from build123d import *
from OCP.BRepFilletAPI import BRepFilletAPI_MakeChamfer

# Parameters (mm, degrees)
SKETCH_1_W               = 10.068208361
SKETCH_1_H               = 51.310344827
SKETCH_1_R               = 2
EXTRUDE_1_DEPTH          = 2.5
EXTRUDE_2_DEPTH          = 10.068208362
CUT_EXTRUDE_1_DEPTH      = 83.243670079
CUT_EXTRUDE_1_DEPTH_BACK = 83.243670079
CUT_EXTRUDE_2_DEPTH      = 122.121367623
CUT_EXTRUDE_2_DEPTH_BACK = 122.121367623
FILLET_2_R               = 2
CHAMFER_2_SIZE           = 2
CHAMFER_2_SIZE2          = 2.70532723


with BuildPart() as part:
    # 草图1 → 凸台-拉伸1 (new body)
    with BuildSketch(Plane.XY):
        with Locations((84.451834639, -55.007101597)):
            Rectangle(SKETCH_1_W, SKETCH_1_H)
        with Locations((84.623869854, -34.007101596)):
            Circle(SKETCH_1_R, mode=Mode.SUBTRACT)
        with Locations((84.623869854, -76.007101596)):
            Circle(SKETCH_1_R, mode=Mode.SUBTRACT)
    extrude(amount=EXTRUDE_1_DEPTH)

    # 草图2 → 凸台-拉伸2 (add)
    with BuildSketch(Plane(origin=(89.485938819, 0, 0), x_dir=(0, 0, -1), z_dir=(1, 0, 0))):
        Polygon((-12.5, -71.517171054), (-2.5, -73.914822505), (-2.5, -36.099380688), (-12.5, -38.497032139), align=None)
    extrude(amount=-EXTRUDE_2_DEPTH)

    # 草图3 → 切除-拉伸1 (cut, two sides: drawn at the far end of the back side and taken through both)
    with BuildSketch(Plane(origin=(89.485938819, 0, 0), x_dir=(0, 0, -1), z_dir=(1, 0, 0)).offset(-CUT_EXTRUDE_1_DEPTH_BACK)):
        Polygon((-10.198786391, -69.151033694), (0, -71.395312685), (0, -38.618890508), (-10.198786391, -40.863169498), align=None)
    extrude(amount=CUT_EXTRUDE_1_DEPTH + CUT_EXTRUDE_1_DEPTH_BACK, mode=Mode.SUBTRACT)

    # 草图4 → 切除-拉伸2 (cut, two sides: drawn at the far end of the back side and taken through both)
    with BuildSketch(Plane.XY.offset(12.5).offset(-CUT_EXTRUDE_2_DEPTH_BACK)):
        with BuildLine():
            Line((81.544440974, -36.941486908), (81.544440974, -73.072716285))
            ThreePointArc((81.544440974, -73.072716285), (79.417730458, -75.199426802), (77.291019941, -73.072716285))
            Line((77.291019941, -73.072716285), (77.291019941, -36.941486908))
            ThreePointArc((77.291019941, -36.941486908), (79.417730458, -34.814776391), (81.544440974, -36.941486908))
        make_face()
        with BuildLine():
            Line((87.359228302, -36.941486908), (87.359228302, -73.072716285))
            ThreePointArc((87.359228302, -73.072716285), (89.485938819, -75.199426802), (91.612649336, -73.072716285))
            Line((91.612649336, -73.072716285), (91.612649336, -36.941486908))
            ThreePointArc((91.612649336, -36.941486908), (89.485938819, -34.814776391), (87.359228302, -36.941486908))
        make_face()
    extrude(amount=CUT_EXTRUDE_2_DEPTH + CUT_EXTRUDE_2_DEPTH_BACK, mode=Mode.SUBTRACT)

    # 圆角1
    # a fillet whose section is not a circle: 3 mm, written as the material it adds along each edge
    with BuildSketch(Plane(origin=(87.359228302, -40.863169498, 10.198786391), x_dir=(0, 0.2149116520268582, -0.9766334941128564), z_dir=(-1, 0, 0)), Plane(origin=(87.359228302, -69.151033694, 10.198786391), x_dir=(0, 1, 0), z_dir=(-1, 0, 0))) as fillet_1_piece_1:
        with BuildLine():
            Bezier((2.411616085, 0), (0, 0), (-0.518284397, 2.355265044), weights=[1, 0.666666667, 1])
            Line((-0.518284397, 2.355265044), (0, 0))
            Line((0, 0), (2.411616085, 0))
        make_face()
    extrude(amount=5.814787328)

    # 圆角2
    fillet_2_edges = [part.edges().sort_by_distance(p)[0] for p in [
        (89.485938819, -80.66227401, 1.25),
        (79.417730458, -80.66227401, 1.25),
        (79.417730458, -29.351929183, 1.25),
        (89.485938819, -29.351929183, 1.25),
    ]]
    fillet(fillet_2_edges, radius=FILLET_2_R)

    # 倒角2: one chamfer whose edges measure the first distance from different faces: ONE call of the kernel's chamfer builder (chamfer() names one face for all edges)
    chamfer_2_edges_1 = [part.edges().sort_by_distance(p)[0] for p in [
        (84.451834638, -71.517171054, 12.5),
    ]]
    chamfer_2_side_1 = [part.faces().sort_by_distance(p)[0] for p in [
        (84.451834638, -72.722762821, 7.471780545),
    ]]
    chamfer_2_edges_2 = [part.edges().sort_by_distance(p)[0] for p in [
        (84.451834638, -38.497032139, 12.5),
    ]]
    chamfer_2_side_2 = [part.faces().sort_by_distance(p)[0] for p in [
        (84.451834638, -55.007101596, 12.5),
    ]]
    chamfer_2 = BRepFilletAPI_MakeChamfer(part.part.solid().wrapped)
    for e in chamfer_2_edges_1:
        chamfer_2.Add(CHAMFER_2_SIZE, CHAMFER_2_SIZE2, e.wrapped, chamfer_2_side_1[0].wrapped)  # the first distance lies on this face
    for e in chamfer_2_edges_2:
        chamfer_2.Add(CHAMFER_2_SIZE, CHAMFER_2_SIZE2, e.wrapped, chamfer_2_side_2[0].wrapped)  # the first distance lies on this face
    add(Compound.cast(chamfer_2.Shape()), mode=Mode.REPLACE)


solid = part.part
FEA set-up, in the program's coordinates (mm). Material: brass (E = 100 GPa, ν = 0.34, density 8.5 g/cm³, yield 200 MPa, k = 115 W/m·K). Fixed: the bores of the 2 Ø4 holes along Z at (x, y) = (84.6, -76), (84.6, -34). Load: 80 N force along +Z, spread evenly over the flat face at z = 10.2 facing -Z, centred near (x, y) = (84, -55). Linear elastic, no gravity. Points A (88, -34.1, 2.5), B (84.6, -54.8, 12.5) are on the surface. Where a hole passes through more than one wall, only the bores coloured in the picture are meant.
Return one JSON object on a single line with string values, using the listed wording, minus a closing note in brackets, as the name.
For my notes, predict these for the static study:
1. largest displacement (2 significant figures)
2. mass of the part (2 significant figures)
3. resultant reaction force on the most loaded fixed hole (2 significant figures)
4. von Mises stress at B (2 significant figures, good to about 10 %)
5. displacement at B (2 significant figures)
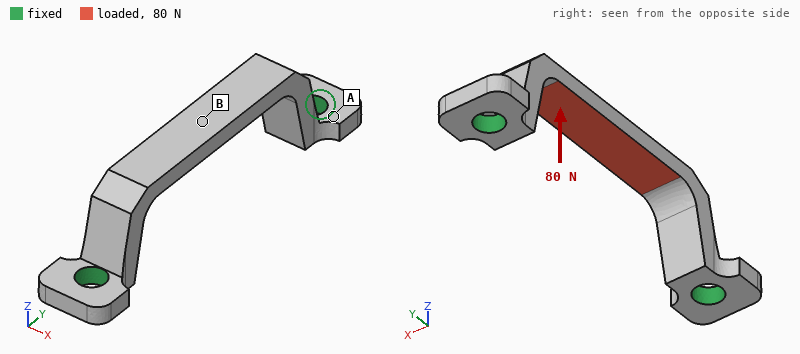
{"largest displacement": "14 µm", "mass of the part": "8.8 g", "resultant reaction force on the most loaded fixed hole": "59 N", "von Mises stress at B": "28 MPa", "displacement at B": "14 µm"}
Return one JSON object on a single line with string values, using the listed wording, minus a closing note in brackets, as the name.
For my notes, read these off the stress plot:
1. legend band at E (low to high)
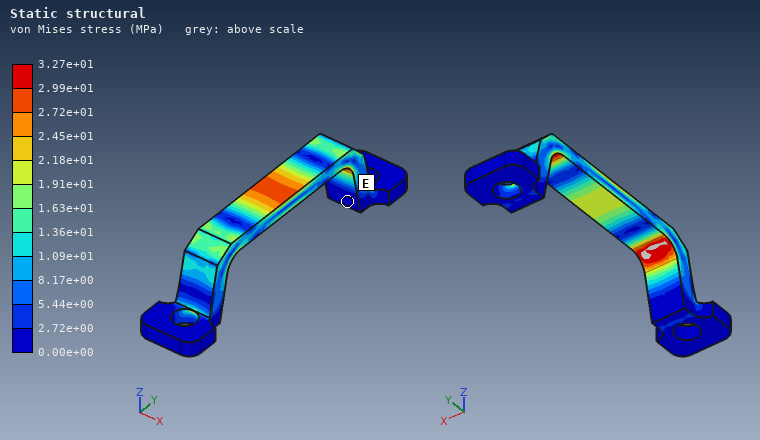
{"legend band at E": "0.00e+00 to 2.72e+00 MPa"}
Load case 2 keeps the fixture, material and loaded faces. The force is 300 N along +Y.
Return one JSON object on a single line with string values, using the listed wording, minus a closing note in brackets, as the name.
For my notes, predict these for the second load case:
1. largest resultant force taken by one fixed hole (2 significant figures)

{"largest resultant force taken by one fixed hole": "150 N"}
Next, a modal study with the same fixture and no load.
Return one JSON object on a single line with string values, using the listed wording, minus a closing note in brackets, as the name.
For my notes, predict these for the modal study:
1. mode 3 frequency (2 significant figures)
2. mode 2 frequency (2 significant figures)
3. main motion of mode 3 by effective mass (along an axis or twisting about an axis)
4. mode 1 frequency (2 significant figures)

{"mode 3 frequency": "8300 Hz", "mode 2 frequency": "7000 Hz", "main motion of mode 3 by effective mass": "along Z", "mode 1 frequency": "6700 Hz"}
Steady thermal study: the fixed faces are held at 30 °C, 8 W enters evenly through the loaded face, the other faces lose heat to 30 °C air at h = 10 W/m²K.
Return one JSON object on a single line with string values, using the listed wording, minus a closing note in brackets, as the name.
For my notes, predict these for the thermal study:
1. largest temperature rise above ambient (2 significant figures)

{"largest temperature rise above ambient": "44 K"}
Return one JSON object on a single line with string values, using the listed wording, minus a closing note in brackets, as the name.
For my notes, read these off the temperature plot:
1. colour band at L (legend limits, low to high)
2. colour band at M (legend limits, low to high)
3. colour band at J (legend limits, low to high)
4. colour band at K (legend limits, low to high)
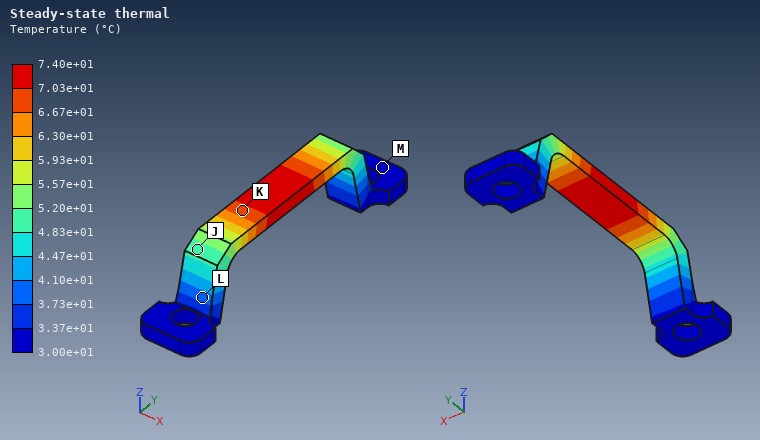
{"colour band at L": "3.73e+01 to 4.10e+01 °C", "colour band at M": "3.00e+01 to 3.37e+01 °C", "colour band at J": "4.83e+01 to 5.20e+01 °C", "colour band at K": "6.67e+01 to 7.03e+01 °C"}
